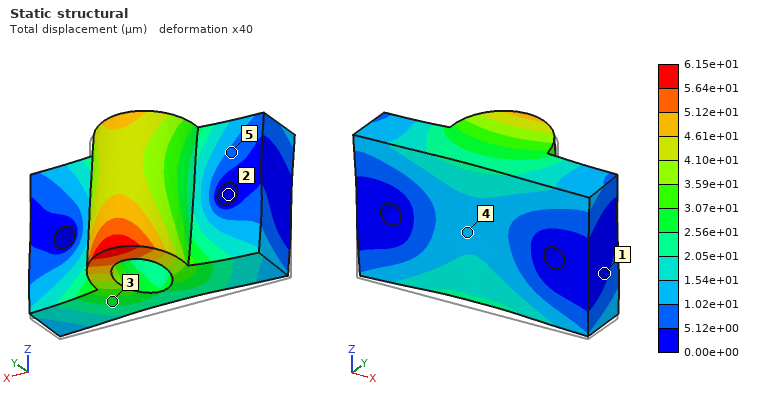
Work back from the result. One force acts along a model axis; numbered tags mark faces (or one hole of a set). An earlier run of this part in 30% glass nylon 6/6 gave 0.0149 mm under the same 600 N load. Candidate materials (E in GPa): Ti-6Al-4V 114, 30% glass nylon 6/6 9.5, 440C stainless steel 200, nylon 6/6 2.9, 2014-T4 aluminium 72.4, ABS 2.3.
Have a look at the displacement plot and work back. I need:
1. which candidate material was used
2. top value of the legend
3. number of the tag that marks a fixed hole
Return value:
ABS
6.15e+01 µm
2
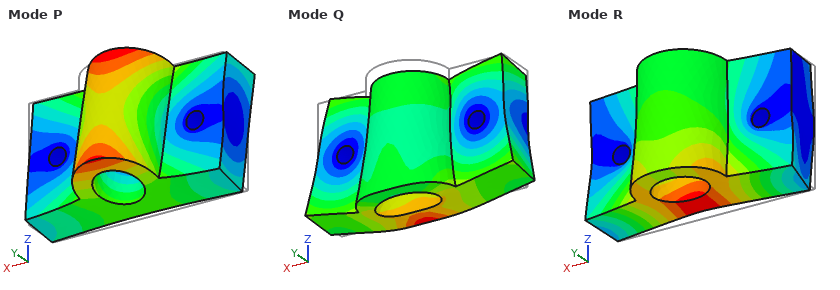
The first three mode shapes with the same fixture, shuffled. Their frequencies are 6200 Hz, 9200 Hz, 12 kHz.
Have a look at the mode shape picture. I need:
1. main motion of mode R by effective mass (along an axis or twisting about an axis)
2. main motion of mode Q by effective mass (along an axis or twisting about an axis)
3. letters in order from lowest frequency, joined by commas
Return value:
along Y
along Z
P, R, Q
